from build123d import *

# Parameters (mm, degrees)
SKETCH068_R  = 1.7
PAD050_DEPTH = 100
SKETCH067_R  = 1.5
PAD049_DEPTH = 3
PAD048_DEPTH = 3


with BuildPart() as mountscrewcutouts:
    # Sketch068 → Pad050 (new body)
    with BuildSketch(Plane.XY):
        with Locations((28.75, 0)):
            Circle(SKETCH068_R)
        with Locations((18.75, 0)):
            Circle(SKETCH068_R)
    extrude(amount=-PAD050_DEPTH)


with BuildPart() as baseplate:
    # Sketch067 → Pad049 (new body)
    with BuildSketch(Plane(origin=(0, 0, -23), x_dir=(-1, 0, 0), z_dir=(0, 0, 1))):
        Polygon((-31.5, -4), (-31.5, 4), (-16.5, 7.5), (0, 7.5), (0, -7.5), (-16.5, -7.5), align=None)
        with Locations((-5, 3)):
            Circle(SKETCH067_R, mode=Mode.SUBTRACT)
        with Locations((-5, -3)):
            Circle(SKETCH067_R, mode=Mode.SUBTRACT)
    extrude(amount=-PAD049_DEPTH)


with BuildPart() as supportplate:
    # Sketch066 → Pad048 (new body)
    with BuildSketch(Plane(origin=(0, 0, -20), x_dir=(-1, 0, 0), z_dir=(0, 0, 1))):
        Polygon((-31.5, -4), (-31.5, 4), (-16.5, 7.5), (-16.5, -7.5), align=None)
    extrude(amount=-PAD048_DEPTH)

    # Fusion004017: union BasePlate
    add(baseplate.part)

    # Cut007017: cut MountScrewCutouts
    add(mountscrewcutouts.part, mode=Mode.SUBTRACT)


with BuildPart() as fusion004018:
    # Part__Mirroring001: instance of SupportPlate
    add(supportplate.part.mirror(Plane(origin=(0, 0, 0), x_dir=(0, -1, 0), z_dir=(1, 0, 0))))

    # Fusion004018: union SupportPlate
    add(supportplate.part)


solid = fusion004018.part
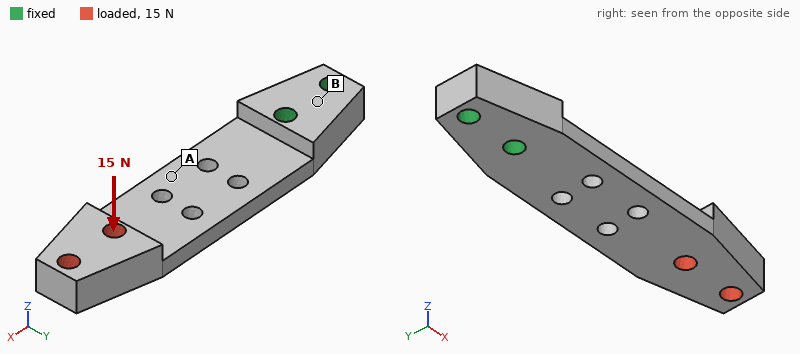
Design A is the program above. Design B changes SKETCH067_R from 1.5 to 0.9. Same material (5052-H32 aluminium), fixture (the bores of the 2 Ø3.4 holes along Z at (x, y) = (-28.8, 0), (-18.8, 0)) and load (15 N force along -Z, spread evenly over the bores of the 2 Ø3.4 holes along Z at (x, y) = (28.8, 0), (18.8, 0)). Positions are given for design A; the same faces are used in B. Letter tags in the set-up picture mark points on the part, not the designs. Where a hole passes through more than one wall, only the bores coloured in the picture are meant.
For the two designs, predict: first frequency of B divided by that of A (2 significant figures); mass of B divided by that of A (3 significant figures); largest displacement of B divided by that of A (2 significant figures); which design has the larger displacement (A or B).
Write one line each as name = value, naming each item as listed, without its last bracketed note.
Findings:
first frequency of B divided by that of A = 1.0
mass of B divided by that of A = 1.02
largest displacement of B divided by that of A = 0.92
which design has the larger displacement = A
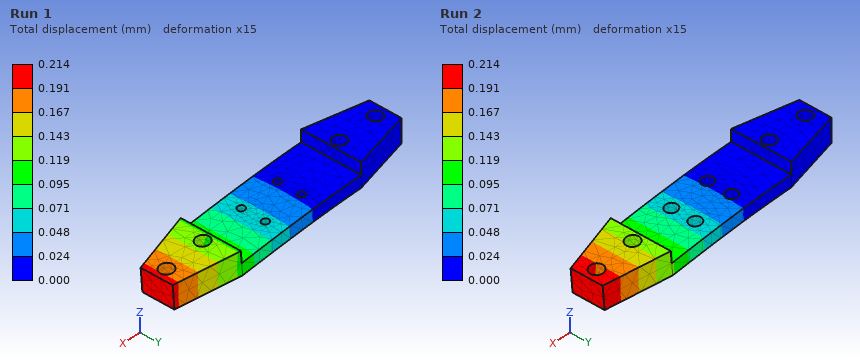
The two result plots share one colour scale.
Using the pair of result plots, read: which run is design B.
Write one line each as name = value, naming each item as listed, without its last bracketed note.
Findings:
which run is design B = Run 1
